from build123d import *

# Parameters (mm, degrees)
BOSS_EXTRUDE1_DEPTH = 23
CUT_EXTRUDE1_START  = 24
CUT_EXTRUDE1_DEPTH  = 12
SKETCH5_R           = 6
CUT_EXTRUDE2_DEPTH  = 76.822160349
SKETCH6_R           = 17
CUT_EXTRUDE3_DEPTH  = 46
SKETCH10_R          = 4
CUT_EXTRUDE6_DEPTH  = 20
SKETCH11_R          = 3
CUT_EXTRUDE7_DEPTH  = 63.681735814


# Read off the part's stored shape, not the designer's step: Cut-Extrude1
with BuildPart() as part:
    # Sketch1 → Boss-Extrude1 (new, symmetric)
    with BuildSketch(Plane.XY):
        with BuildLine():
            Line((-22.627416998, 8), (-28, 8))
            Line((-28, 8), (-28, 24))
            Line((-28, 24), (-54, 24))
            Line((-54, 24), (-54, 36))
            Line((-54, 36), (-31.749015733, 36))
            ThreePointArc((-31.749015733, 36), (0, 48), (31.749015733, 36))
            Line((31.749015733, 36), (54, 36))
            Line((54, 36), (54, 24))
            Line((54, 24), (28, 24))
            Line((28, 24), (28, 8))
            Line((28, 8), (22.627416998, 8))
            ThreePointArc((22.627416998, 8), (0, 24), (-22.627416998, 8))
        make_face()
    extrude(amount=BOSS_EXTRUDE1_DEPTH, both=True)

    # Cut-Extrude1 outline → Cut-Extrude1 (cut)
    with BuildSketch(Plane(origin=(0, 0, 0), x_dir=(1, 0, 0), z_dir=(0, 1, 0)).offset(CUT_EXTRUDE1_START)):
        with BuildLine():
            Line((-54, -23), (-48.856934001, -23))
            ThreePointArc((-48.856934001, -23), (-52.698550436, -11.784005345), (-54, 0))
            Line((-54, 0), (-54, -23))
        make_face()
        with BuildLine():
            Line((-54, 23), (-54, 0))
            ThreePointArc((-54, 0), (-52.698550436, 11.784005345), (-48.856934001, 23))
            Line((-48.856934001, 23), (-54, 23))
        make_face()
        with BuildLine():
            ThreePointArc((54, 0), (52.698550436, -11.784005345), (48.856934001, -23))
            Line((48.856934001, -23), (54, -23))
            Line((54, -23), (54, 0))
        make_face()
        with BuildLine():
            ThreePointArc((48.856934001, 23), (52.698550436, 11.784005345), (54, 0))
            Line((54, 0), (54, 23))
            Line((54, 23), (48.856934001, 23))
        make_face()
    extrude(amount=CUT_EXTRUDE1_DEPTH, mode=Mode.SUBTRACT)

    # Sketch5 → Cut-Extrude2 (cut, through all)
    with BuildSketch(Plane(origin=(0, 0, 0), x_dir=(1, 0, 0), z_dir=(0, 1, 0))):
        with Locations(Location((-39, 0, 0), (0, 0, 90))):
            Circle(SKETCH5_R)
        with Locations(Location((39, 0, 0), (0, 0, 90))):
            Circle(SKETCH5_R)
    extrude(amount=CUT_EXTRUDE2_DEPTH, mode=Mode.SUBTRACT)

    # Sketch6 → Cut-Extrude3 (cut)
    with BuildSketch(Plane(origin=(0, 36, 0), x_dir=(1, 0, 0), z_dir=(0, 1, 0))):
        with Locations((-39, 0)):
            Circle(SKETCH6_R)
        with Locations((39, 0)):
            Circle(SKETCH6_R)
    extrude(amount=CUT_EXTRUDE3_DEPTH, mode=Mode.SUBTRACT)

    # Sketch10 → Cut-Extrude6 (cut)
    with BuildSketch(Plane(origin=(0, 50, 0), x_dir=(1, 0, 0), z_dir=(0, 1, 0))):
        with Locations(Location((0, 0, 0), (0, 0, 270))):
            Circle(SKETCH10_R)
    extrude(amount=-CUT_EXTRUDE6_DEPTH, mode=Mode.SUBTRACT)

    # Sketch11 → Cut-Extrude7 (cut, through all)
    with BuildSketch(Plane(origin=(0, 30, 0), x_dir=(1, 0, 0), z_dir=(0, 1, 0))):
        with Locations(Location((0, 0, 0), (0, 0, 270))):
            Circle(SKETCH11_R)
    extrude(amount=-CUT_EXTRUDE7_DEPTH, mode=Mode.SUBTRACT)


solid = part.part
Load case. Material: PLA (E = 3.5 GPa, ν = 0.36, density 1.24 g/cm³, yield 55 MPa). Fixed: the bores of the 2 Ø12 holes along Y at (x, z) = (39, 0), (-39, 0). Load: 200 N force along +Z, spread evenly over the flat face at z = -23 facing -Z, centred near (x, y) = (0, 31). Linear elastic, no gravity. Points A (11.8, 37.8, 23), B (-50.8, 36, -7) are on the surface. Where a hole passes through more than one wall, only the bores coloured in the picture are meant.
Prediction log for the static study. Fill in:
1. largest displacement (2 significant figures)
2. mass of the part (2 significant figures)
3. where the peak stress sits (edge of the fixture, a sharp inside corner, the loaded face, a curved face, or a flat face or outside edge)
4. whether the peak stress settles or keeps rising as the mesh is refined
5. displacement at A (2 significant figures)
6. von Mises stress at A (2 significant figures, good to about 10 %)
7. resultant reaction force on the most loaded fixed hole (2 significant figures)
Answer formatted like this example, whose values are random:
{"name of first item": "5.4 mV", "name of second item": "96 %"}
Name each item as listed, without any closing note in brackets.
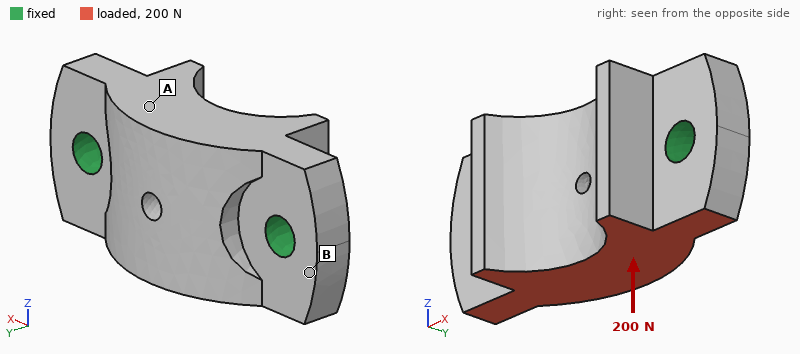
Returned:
{"largest displacement": "5.2 µm", "mass of the part": "120 g", "where the peak stress sits": "edge of the fixture", "whether the peak stress settles or keeps rising as the mesh is refined": "keeps rising", "displacement at A": "3.4 µm", "von Mises stress at A": "0.16 MPa", "resultant reaction force on the most loaded fixed hole": "100 N"}
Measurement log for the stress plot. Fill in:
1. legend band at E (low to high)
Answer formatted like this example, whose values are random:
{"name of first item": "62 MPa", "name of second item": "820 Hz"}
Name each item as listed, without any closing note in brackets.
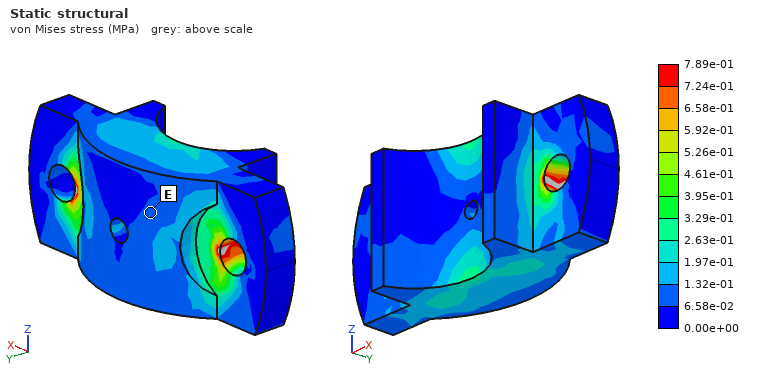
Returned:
{"legend band at E": "6.58e-02 to 1.32e-01 MPa"}
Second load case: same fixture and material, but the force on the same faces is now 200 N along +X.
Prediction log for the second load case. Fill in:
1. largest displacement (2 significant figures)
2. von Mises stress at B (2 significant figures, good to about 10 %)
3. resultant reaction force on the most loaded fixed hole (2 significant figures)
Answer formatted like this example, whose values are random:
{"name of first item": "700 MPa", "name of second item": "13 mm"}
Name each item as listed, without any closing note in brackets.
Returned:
{"largest displacement": "5.1 µm", "von Mises stress at B": "0.18 MPa", "resultant reaction force on the most loaded fixed hole": "110 N"}
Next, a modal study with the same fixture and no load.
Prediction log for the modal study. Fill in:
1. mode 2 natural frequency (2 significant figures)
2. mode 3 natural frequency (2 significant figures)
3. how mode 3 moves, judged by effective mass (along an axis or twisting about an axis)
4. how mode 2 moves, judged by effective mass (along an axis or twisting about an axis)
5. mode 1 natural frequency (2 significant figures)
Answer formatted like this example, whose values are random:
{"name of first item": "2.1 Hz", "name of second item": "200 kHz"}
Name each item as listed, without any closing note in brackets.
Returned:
{"mode 2 natural frequency": "3000 Hz", "mode 3 natural frequency": "3900 Hz", "how mode 3 moves, judged by effective mass": "along Z", "how mode 2 moves, judged by effective mass": "along Y", "mode 1 natural frequency": "2500 Hz"}
